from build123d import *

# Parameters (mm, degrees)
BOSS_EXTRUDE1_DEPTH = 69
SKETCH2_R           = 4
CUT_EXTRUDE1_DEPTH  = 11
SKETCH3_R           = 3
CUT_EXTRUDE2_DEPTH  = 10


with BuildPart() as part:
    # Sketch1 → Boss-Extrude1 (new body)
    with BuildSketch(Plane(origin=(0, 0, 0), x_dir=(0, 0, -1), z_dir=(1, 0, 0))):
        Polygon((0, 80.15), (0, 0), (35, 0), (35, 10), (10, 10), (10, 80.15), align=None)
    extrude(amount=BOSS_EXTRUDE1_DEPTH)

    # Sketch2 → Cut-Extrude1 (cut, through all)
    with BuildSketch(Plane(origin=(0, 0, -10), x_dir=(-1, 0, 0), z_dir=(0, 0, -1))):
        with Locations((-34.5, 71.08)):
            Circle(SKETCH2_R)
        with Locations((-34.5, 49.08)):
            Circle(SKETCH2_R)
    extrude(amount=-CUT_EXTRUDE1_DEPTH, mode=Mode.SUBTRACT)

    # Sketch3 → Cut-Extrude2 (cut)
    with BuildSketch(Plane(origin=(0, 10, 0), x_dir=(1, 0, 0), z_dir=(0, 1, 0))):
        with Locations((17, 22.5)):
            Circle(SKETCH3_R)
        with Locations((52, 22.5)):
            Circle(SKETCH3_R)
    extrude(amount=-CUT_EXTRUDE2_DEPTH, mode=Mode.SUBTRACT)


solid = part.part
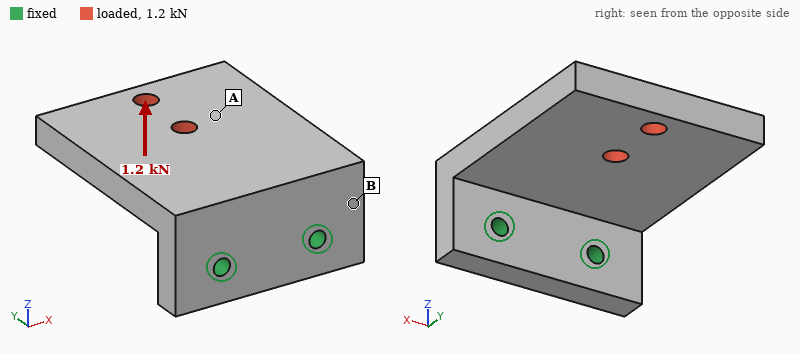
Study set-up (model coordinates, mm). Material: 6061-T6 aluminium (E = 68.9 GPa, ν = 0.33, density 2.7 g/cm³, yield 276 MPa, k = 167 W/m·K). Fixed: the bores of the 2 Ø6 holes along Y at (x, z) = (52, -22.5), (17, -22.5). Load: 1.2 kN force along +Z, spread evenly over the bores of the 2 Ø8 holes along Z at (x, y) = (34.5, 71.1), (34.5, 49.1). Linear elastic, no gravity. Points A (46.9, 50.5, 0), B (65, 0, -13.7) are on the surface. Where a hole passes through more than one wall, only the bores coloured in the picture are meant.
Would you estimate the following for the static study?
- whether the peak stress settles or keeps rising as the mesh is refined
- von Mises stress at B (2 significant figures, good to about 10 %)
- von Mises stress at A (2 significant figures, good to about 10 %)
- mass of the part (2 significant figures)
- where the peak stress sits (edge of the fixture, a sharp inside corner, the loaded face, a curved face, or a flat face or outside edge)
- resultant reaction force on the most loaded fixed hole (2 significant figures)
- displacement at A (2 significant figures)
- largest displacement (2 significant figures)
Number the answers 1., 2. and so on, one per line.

1. keeps rising
2. 46 MPa
3. 13 MPa
4. 190 g
5. edge of the fixture
6. 660 N
7. 0.25 mm
8. 0.47 mm
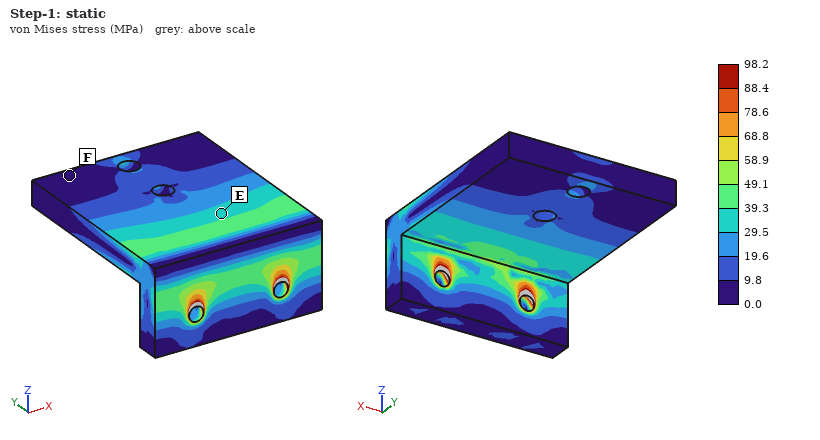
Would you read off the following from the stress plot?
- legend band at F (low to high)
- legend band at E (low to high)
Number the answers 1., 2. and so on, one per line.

1. 0.0 to 9.8 MPa
2. 29.5 to 39.3 MPa
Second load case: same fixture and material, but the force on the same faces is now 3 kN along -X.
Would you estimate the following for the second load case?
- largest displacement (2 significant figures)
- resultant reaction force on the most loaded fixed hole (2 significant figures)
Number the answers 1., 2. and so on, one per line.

1. 0.16 mm
2. 4.3 kN
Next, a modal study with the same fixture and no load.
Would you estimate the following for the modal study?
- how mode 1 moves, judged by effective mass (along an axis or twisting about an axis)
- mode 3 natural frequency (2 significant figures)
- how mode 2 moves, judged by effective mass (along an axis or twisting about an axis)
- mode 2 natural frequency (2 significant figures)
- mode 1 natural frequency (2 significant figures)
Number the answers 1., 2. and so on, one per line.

1. along Z
2. 3500 Hz
3. along X
4. 2600 Hz
5. 1100 Hz
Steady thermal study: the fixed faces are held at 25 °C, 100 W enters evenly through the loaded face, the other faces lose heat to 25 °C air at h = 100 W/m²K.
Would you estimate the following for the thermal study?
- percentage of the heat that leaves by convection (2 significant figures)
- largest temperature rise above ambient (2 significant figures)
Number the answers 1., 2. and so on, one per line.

1. 39 %
2. 52 K
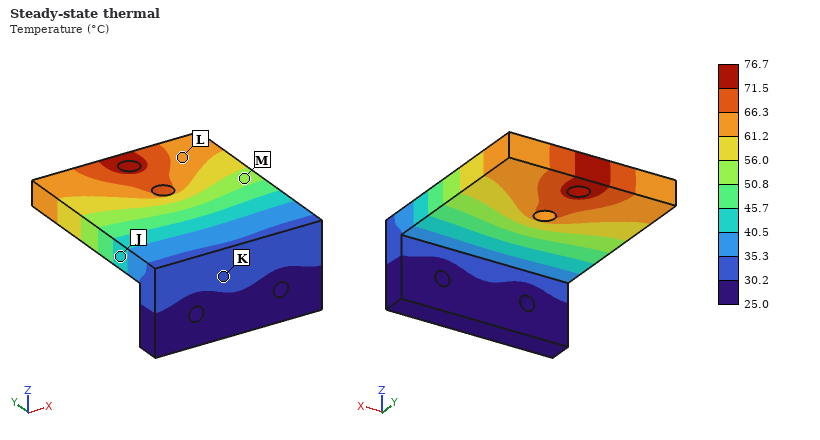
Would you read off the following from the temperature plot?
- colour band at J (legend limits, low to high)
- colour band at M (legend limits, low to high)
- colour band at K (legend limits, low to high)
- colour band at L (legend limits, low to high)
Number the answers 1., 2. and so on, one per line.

1. 40.5 to 45.7 °C
2. 50.8 to 56.0 °C
3. 30.2 to 35.3 °C
4. 61.2 to 66.3 °C
